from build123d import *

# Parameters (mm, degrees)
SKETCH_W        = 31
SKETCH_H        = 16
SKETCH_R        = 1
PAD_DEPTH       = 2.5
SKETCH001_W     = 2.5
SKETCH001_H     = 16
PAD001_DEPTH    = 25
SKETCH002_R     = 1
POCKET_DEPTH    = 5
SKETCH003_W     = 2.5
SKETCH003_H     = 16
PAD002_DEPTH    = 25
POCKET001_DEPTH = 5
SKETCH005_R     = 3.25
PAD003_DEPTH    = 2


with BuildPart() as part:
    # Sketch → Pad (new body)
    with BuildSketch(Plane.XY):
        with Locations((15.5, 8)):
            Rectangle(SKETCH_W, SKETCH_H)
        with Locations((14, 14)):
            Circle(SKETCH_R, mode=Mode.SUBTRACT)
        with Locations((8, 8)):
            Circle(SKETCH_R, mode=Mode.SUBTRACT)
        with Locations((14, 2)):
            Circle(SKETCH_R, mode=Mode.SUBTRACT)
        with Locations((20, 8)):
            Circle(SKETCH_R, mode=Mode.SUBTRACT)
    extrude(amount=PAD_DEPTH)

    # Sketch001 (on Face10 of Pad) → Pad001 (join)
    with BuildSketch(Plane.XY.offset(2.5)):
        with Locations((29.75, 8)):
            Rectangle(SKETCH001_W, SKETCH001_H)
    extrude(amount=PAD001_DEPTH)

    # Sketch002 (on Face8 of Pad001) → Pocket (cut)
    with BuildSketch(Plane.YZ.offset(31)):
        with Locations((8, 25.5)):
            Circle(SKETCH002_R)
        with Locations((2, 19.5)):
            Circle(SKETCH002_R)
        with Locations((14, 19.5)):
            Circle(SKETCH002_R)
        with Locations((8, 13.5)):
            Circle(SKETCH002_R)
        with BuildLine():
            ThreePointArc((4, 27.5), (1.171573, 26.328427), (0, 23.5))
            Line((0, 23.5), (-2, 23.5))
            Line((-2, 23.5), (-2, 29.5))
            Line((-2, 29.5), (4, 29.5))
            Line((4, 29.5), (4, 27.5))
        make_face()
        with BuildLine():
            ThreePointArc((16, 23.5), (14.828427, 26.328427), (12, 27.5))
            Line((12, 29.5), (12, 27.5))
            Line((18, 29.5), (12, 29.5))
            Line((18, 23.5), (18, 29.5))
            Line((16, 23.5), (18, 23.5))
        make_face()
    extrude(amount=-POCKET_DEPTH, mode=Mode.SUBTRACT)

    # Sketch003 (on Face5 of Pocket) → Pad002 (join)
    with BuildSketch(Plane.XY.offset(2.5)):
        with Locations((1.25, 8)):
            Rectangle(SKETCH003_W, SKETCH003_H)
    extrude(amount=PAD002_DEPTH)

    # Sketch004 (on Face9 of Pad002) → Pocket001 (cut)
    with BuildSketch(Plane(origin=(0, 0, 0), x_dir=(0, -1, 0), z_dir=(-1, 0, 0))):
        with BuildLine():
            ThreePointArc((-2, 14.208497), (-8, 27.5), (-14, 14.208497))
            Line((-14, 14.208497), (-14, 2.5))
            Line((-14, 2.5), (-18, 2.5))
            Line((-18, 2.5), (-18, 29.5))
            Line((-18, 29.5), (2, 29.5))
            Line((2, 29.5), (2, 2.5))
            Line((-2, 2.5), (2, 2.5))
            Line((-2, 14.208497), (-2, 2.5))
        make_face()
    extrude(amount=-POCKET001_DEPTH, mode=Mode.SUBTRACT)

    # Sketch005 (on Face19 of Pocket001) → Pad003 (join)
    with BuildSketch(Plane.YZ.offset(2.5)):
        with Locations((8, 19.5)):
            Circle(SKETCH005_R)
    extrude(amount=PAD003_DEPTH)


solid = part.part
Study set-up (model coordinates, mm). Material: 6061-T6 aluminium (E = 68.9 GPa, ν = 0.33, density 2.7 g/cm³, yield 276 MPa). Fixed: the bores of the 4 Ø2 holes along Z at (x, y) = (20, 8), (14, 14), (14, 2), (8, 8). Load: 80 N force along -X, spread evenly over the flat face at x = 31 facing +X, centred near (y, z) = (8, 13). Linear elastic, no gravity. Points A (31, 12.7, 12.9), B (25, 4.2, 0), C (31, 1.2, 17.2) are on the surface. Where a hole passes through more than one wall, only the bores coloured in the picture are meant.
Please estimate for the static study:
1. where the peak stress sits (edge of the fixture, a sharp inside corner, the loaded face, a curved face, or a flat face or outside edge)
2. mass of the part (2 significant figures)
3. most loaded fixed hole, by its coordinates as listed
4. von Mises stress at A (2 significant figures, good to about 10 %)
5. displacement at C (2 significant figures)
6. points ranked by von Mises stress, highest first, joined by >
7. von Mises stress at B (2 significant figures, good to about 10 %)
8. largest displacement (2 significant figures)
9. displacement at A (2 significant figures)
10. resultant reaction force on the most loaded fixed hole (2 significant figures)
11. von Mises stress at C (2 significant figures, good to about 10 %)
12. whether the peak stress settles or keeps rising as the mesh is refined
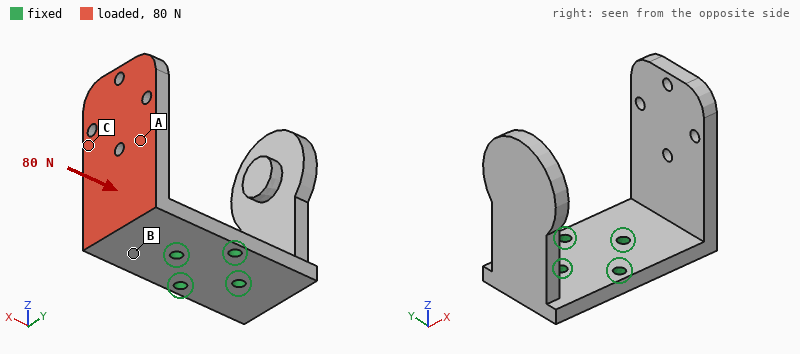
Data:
edge of the fixture
8.2 g
(20, 8)
19 MPa
0.16 mm
B > A > C
50 MPa
0.27 mm
0.11 mm
99 N
8.9 MPa
keeps rising
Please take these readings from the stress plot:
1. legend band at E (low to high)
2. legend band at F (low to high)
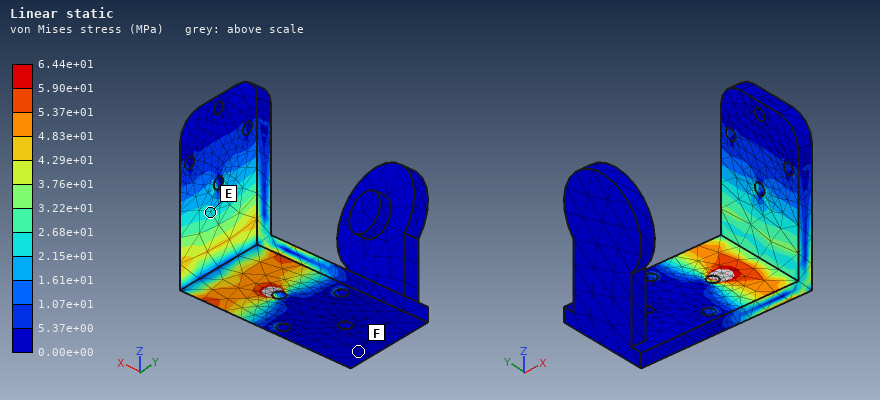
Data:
2.15e+01 to 2.68e+01 MPa
0.00e+00 to 5.37e+00 MPa
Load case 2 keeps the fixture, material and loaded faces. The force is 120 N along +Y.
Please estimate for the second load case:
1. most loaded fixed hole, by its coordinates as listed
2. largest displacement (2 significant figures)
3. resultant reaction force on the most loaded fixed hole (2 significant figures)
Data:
(20, 8)
0.16 mm
140 N
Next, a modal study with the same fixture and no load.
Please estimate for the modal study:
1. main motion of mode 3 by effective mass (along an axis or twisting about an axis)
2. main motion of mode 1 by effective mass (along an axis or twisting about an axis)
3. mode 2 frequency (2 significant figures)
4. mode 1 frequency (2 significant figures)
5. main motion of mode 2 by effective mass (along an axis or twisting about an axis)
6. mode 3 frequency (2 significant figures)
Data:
along Y
along X
2100 Hz
2000 Hz
along X
3100 Hz
